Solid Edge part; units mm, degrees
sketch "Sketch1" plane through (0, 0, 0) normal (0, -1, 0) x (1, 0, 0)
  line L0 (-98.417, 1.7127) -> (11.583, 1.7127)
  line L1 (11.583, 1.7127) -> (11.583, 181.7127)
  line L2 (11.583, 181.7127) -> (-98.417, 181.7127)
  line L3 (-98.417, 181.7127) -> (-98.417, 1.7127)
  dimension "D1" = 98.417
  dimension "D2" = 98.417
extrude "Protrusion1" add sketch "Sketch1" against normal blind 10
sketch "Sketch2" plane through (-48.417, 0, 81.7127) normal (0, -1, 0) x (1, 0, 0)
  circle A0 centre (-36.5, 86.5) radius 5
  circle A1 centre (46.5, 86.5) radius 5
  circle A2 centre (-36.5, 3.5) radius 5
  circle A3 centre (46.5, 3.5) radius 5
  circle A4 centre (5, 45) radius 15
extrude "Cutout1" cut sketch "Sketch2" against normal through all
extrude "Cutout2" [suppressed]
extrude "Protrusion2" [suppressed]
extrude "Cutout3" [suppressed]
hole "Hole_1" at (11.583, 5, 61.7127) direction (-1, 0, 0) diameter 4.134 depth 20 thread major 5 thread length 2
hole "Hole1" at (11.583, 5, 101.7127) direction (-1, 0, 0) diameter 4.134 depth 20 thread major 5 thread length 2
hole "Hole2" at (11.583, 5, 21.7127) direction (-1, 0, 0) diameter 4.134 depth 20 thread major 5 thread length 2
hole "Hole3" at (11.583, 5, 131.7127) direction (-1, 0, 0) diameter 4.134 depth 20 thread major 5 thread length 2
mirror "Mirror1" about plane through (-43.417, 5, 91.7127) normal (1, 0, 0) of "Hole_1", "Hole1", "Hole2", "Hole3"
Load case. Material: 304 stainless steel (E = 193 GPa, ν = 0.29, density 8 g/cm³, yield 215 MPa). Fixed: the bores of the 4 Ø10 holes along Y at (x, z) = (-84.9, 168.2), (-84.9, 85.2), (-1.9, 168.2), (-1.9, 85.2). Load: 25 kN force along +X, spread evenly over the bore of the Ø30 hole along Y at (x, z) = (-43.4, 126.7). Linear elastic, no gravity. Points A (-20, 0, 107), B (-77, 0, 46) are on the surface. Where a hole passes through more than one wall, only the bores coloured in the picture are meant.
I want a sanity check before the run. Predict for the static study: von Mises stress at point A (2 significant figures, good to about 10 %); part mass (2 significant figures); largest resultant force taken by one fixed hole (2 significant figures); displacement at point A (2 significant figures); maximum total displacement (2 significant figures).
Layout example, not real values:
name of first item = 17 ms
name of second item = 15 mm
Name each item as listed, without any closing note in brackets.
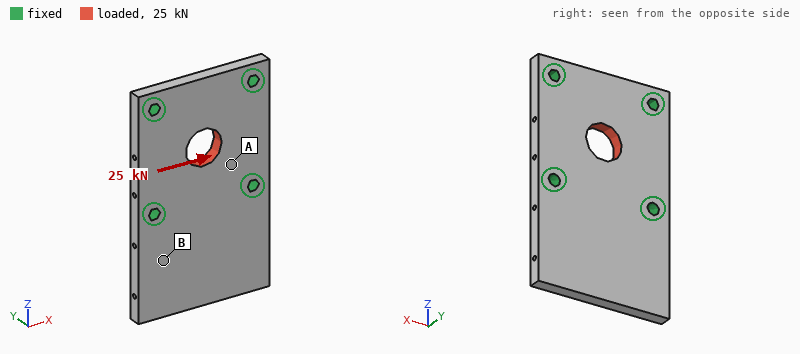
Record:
von Mises stress at point A = 24 MPa
part mass = 1.5 kg
largest resultant force taken by one fixed hole = 6.9 kN
displacement at point A = 4.6 µm
maximum total displacement = 7.9 µm
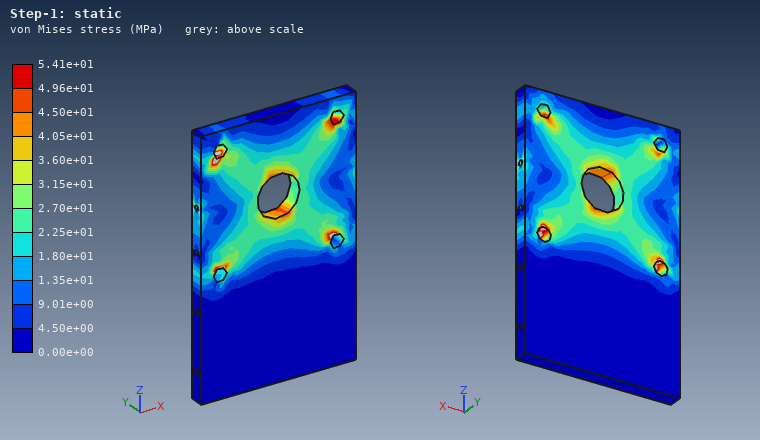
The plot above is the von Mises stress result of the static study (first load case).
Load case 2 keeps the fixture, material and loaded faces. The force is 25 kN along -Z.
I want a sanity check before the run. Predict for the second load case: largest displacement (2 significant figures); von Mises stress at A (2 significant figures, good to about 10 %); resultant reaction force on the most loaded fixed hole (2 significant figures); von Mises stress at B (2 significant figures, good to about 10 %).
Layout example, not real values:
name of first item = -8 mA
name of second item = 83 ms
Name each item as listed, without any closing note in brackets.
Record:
largest displacement = 7.7 µm
von Mises stress at A = 22 MPa
resultant reaction force on the most loaded fixed hole = 7.0 kN
von Mises stress at B = 4.0 MPa
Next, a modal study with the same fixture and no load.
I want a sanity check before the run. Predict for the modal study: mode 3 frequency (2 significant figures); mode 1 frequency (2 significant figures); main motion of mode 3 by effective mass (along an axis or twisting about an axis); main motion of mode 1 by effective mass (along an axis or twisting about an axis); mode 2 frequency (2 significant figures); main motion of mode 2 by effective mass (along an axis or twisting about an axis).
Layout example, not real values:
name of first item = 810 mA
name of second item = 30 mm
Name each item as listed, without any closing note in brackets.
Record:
mode 3 frequency = 5200 Hz
mode 1 frequency = 1100 Hz
main motion of mode 3 by effective mass = along Y
main motion of mode 1 by effective mass = along Y
mode 2 frequency = 2300 Hz
main motion of mode 2 by effective mass = twisting about Z
